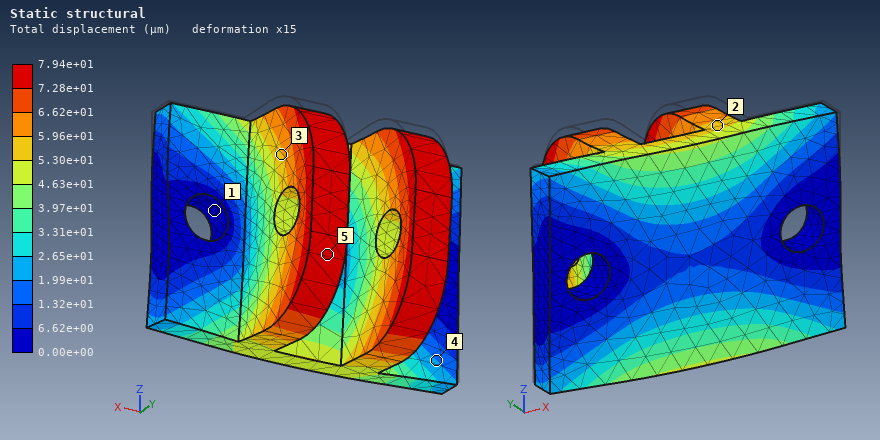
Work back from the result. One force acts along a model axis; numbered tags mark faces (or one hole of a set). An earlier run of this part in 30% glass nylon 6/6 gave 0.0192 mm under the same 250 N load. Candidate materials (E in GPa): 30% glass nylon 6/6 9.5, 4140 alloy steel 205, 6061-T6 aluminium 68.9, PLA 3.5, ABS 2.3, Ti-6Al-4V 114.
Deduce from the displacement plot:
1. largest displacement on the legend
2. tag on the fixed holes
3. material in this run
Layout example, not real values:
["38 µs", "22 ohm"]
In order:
["7.94e+01 µm", "1", "ABS"]
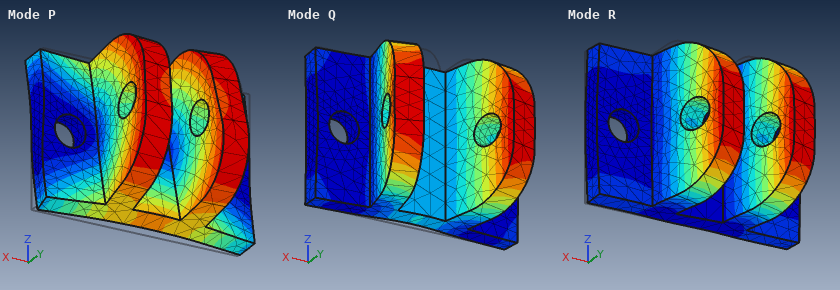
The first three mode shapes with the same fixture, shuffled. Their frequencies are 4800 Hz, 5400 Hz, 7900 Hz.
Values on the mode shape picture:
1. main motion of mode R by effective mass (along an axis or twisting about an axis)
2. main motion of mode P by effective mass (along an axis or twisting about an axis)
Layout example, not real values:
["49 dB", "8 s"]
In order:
["along X", "along Z"]
